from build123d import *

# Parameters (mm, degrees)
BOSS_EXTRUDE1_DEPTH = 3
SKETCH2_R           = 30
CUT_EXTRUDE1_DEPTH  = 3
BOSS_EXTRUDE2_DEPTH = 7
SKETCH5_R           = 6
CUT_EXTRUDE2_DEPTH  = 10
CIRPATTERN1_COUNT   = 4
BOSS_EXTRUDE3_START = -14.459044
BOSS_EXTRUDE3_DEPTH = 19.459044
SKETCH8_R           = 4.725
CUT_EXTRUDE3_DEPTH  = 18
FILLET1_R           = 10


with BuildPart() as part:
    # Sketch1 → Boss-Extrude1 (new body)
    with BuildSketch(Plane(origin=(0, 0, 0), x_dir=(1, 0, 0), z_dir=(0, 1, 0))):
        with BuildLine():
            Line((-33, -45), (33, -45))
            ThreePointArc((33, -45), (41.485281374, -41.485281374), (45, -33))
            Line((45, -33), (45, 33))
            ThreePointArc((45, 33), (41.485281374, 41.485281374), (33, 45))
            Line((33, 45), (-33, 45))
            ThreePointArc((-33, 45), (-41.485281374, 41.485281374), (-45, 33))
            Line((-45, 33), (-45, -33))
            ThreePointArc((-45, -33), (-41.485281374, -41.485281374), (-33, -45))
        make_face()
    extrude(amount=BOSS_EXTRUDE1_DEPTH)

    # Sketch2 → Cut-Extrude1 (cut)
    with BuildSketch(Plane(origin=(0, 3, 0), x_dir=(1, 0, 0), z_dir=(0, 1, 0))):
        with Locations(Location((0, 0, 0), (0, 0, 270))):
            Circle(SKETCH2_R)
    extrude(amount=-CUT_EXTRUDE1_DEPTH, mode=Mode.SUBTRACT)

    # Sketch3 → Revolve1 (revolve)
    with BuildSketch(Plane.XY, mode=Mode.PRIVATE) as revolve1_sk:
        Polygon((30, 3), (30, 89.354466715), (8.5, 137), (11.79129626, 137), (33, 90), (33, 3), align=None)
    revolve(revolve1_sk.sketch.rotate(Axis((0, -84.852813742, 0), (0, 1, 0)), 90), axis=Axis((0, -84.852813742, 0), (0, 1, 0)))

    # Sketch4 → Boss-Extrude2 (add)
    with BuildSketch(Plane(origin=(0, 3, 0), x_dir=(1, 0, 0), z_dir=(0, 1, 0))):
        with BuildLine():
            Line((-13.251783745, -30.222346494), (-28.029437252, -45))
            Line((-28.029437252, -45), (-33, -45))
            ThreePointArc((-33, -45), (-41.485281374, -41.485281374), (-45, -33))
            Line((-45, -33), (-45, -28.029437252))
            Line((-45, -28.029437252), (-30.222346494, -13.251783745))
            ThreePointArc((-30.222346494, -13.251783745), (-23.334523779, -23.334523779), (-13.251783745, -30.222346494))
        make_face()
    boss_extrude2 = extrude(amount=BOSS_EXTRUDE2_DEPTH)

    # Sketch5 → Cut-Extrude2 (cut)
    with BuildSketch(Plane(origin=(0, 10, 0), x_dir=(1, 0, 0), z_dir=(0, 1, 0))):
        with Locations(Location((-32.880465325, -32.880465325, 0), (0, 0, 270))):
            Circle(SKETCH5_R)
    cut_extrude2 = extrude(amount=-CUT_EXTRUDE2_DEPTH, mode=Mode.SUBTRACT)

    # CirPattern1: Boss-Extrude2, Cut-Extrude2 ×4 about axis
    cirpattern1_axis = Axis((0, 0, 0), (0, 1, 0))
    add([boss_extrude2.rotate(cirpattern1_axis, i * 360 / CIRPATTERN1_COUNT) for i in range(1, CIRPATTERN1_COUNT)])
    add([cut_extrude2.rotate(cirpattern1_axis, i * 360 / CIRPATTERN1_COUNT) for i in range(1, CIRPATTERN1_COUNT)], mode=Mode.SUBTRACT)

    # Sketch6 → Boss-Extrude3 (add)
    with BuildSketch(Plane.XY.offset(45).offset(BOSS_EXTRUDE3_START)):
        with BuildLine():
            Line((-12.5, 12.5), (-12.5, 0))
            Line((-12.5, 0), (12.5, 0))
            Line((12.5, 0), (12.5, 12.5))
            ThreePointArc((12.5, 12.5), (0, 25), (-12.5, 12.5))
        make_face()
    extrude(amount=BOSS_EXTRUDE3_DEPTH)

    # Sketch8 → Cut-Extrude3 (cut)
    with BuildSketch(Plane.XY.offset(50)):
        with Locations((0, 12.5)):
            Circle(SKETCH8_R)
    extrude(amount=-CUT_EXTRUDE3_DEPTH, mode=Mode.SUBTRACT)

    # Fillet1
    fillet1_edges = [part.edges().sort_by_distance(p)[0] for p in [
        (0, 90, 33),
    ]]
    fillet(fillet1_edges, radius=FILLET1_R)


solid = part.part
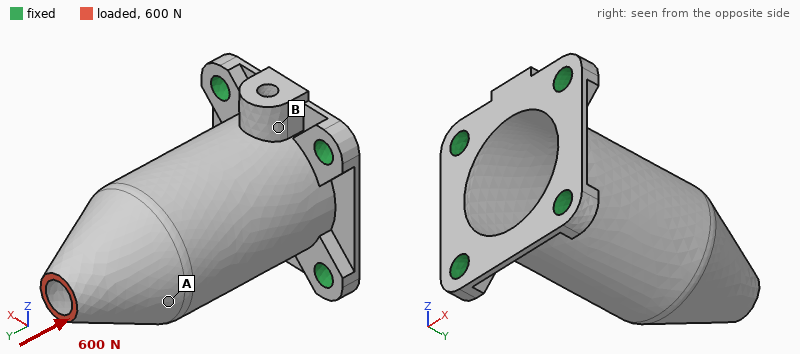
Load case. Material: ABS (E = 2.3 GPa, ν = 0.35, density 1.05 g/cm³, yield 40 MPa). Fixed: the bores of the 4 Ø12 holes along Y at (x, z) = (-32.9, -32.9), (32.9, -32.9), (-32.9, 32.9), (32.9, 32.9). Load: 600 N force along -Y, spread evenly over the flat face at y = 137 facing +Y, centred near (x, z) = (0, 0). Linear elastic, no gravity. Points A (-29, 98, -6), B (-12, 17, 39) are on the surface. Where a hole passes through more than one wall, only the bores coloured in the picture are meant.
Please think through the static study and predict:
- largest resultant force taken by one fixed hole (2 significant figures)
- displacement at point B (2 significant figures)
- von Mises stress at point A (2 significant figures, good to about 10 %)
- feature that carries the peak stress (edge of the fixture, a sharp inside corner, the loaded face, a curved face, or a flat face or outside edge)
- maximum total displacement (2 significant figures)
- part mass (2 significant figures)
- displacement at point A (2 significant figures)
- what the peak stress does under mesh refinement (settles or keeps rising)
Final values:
150 N
0.026 mm
1.6 MPa
a sharp inside corner
0.14 mm
110 g
0.069 mm
keeps rising
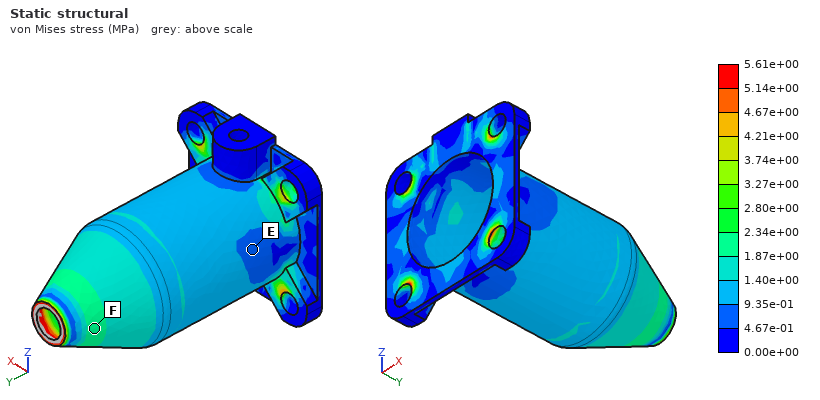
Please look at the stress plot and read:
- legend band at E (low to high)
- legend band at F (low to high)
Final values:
4.67e-01 to 9.35e-01 MPa
1.87e+00 to 2.34e+00 MPa
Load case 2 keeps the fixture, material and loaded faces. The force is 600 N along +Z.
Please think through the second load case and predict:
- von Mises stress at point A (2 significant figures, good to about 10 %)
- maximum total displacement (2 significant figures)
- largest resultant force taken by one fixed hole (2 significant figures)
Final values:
2.2 MPa
1.7 mm
760 N
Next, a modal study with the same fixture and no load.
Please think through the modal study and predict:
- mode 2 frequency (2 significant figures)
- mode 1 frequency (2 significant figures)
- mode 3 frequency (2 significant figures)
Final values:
690 Hz
670 Hz
1500 Hz
